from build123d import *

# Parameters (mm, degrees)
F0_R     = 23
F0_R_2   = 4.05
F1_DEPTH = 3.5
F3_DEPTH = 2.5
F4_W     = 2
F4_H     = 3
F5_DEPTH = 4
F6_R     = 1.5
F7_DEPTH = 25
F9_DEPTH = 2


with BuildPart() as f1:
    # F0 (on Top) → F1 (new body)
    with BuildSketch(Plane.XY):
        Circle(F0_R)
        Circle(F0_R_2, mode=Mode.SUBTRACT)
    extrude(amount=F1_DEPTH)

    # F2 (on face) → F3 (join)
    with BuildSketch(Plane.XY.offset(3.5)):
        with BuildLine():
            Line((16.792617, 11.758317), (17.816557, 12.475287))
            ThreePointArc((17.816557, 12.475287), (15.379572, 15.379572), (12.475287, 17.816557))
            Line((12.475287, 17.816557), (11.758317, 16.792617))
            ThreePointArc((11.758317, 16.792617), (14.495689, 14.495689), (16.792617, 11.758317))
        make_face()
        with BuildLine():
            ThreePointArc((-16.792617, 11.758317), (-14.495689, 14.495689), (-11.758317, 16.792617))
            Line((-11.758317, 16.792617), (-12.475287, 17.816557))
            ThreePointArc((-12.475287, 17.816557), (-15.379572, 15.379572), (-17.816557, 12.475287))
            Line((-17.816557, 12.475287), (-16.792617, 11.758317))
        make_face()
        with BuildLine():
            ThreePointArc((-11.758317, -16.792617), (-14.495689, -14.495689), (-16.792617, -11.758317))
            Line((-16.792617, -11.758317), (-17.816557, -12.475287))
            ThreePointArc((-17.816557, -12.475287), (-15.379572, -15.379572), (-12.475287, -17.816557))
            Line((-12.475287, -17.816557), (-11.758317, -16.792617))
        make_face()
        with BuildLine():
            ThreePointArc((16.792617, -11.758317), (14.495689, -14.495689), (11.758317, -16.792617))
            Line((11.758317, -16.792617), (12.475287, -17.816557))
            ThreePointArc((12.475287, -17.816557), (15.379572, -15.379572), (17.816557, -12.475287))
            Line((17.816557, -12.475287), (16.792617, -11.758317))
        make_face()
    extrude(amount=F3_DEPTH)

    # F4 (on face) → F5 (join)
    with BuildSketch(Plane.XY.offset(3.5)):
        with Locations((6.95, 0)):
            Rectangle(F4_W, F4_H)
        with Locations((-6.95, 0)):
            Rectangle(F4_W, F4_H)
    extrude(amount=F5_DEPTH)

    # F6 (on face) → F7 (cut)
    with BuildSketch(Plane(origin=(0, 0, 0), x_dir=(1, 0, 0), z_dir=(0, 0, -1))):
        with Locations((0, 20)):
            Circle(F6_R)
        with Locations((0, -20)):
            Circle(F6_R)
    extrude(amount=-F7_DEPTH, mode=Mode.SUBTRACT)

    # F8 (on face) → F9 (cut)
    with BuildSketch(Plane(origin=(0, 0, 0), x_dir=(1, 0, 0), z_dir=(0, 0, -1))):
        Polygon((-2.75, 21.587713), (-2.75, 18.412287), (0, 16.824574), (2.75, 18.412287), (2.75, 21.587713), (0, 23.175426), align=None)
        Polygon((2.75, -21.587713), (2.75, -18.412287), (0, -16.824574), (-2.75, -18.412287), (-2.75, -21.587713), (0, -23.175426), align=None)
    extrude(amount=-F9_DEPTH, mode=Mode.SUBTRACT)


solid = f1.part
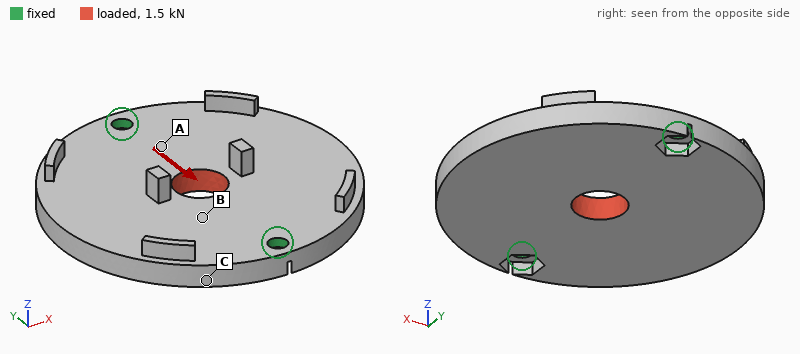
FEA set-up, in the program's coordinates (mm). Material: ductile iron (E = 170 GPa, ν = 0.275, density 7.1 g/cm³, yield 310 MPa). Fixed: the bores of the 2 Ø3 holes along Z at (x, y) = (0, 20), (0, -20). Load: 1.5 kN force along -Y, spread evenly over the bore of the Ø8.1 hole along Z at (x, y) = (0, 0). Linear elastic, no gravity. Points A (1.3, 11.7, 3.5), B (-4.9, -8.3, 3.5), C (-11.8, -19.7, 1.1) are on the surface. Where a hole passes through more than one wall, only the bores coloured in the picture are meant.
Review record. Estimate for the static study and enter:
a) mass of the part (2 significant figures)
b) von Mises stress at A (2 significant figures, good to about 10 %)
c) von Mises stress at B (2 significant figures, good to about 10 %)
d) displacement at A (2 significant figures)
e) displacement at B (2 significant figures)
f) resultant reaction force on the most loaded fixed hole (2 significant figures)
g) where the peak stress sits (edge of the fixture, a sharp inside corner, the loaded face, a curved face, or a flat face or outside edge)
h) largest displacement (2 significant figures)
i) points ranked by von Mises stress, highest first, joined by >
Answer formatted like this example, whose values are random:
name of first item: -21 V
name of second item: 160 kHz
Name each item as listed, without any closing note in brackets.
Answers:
mass of the part: 40 g
von Mises stress at A: 26 MPa
von Mises stress at B: 16 MPa
displacement at A: 2.0 µm
displacement at B: 2.3 µm
resultant reaction force on the most loaded fixed hole: 750 N
where the peak stress sits: edge of the fixture
largest displacement: 3.0 µm
points ranked by von Mises stress, highest first, joined by >: A > B > C
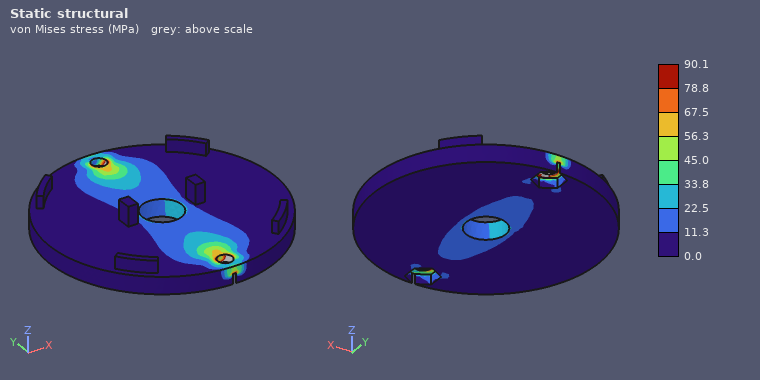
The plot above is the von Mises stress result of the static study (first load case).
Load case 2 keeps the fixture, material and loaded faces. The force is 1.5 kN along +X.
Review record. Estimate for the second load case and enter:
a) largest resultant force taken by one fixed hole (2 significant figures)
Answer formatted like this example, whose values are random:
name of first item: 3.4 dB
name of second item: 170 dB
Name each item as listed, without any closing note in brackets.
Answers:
largest resultant force taken by one fixed hole: 750 N
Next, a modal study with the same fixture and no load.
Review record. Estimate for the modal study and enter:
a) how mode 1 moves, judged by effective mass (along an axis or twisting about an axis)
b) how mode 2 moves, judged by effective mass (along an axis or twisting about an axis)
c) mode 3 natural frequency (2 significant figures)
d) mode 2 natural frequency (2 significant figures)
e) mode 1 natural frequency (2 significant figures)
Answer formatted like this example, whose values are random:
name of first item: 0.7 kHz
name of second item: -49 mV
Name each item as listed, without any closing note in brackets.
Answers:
how mode 1 moves, judged by effective mass: twisting about Y
how mode 2 moves, judged by effective mass: along Z
mode 3 natural frequency: 9400 Hz
mode 2 natural frequency: 4500 Hz
mode 1 natural frequency: 2300 Hz
